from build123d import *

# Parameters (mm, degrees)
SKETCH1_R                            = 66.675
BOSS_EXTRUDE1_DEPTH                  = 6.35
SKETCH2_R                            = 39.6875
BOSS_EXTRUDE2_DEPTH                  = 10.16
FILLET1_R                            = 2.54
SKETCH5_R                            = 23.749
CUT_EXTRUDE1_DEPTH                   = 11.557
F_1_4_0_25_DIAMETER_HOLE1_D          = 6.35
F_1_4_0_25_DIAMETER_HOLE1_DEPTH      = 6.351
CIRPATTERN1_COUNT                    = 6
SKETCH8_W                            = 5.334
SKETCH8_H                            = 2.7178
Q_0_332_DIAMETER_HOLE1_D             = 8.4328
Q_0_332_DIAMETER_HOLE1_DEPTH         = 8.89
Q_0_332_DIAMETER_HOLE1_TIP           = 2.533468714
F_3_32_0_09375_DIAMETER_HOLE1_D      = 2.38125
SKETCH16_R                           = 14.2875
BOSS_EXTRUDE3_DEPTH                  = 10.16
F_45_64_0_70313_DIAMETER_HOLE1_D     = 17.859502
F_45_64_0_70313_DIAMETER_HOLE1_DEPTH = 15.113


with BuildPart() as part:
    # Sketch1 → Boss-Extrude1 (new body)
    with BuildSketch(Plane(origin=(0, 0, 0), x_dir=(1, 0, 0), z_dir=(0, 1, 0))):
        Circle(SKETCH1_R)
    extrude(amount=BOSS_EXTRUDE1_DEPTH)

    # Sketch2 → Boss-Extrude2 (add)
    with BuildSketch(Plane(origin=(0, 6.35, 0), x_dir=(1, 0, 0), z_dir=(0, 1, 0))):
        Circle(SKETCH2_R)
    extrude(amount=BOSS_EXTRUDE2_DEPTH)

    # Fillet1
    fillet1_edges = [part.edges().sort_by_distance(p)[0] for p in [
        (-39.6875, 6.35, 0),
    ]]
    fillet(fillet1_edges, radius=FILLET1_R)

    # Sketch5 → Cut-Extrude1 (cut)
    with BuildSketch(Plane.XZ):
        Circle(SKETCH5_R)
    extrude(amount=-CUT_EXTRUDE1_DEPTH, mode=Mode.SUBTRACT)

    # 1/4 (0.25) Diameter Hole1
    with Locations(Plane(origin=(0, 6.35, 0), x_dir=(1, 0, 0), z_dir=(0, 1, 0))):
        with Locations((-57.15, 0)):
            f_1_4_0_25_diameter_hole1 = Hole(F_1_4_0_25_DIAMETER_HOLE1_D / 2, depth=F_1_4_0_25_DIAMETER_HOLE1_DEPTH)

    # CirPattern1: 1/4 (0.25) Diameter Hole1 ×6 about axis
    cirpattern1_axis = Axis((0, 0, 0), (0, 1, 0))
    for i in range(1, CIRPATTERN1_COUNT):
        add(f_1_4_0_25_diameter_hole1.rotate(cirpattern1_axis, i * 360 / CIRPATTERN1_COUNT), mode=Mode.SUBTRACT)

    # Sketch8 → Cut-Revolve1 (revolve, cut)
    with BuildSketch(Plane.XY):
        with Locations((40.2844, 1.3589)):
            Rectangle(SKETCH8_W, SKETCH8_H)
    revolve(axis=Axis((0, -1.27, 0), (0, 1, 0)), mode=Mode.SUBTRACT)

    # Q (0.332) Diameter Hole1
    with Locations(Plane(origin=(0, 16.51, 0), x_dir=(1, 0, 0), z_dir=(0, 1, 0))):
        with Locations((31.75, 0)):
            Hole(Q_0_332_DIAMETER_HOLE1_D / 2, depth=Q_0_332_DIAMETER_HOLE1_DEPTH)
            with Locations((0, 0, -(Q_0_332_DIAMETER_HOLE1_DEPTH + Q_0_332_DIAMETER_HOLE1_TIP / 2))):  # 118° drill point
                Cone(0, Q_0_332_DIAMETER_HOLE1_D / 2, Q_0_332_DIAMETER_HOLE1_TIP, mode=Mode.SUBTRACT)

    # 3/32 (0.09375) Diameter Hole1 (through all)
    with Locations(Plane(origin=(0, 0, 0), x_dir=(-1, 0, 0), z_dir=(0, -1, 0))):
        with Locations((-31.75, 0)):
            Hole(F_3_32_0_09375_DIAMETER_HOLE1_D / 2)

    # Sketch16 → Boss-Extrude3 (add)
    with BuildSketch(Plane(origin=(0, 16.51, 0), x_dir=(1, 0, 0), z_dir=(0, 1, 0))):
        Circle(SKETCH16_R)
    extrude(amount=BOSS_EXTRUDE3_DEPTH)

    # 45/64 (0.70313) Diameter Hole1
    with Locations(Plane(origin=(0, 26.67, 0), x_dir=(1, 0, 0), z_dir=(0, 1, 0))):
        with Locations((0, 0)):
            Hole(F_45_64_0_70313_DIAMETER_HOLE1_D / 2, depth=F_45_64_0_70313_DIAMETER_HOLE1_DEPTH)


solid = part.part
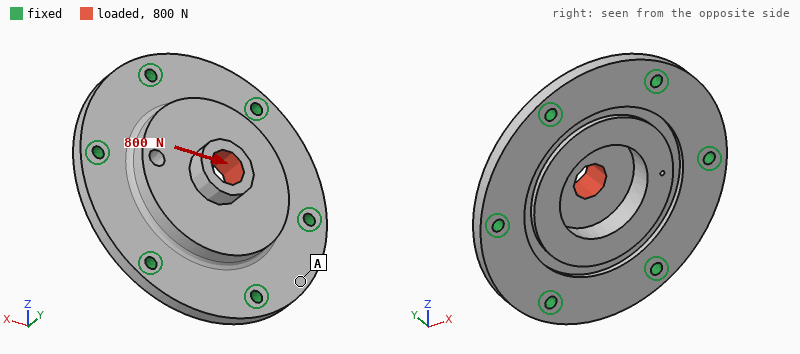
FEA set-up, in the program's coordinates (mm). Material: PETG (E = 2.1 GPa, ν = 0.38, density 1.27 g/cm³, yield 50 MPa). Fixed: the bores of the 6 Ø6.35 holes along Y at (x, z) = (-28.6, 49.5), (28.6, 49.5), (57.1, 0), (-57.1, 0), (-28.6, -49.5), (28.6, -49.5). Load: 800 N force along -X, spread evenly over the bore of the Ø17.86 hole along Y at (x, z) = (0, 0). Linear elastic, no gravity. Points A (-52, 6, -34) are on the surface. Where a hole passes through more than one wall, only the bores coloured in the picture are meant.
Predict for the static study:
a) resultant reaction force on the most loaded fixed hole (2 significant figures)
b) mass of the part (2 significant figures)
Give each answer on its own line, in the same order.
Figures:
220 N
150 g
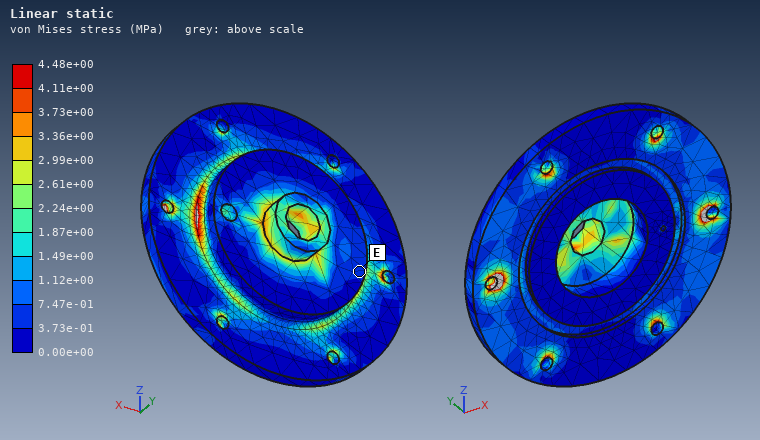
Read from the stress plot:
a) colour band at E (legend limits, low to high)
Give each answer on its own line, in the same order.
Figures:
3.73e-01 to 7.47e-01 MPa
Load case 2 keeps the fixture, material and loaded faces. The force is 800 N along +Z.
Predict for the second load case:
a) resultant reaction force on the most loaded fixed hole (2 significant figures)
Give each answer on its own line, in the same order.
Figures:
190 N
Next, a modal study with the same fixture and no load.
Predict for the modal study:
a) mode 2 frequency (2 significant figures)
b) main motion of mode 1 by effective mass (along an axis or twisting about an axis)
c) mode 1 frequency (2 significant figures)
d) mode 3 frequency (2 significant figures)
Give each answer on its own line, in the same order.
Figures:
1900 Hz
along Y
1400 Hz
1900 Hz
